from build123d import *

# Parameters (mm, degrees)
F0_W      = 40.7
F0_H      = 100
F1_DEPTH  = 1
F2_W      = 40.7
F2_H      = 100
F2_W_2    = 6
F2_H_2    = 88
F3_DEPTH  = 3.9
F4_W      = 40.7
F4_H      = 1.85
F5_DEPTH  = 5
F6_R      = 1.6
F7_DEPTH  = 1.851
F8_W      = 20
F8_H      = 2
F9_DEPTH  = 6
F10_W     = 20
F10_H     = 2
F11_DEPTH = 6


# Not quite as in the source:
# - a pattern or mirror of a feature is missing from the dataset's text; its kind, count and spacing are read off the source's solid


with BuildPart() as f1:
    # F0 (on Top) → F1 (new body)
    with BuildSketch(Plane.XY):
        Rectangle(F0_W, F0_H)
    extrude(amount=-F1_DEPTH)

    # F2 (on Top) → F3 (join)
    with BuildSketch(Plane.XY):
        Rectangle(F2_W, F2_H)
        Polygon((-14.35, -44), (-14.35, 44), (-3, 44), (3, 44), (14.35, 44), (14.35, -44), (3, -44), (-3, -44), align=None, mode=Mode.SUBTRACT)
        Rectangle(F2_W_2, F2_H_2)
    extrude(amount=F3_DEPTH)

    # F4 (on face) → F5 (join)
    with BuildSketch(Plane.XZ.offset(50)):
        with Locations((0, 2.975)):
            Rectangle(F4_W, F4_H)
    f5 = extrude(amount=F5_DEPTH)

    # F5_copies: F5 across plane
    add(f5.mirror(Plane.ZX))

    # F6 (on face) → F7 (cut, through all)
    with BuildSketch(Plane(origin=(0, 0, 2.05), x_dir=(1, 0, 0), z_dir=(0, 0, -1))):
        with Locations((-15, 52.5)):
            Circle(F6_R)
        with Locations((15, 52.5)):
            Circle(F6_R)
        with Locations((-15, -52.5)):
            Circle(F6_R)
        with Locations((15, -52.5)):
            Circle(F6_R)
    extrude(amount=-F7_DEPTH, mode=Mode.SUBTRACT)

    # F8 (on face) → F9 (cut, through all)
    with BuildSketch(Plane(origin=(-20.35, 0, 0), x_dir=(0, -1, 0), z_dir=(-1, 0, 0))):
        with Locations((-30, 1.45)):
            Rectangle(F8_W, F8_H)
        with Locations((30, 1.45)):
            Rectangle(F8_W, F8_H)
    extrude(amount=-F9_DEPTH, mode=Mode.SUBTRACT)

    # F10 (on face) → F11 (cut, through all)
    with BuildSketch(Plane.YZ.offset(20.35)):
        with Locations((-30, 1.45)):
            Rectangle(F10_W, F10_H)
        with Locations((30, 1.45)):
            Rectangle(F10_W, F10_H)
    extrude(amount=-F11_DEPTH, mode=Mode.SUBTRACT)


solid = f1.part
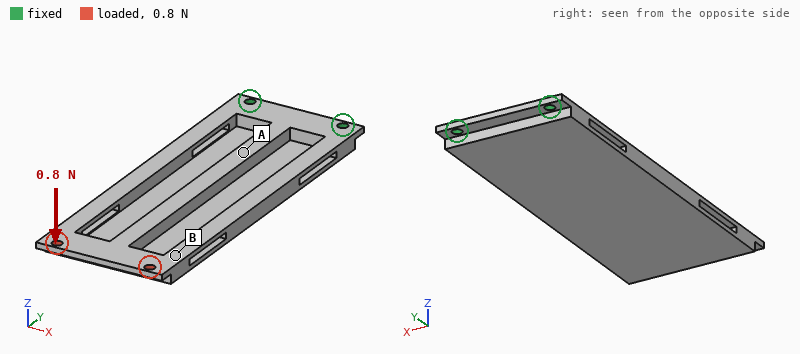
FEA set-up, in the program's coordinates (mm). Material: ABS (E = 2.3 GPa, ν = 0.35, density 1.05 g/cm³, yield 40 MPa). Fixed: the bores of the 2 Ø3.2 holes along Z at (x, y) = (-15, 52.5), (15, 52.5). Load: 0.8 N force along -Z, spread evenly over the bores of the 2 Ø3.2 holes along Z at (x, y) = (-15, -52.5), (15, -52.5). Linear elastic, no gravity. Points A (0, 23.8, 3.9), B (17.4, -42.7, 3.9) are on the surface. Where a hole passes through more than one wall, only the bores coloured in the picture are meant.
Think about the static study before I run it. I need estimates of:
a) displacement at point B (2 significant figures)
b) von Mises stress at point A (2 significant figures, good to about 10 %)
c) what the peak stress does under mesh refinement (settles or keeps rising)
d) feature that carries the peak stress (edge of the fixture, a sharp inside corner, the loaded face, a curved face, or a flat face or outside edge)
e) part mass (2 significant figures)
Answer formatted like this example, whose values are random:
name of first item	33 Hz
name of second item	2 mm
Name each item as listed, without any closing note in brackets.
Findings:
displacement at point B	1.1 mm
von Mises stress at point A	0.72 MPa
what the peak stress does under mesh refinement	keeps rising
feature that carries the peak stress	edge of the fixture
part mass	12 g
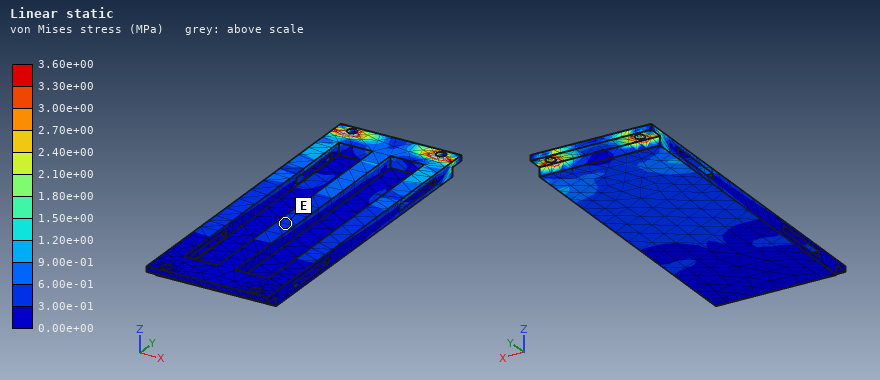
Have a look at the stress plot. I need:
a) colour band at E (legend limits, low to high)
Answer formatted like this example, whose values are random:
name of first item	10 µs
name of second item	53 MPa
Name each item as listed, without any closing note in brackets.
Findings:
colour band at E	3.00e-01 to 6.00e-01 MPa
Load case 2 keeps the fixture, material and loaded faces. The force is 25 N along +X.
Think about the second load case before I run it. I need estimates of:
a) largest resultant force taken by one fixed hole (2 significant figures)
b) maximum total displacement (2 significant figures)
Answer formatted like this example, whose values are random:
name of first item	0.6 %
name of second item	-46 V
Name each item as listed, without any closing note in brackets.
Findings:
largest resultant force taken by one fixed hole	84 N
maximum total displacement	1.2 mm
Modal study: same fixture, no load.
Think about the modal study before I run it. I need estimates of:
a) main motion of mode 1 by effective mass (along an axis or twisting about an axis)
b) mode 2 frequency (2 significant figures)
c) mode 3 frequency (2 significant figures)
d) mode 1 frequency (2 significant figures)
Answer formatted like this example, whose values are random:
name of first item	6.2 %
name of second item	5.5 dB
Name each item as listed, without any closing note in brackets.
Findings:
main motion of mode 1 by effective mass	along Z
mode 2 frequency	270 Hz
mode 3 frequency	470 Hz
mode 1 frequency	65 Hz
